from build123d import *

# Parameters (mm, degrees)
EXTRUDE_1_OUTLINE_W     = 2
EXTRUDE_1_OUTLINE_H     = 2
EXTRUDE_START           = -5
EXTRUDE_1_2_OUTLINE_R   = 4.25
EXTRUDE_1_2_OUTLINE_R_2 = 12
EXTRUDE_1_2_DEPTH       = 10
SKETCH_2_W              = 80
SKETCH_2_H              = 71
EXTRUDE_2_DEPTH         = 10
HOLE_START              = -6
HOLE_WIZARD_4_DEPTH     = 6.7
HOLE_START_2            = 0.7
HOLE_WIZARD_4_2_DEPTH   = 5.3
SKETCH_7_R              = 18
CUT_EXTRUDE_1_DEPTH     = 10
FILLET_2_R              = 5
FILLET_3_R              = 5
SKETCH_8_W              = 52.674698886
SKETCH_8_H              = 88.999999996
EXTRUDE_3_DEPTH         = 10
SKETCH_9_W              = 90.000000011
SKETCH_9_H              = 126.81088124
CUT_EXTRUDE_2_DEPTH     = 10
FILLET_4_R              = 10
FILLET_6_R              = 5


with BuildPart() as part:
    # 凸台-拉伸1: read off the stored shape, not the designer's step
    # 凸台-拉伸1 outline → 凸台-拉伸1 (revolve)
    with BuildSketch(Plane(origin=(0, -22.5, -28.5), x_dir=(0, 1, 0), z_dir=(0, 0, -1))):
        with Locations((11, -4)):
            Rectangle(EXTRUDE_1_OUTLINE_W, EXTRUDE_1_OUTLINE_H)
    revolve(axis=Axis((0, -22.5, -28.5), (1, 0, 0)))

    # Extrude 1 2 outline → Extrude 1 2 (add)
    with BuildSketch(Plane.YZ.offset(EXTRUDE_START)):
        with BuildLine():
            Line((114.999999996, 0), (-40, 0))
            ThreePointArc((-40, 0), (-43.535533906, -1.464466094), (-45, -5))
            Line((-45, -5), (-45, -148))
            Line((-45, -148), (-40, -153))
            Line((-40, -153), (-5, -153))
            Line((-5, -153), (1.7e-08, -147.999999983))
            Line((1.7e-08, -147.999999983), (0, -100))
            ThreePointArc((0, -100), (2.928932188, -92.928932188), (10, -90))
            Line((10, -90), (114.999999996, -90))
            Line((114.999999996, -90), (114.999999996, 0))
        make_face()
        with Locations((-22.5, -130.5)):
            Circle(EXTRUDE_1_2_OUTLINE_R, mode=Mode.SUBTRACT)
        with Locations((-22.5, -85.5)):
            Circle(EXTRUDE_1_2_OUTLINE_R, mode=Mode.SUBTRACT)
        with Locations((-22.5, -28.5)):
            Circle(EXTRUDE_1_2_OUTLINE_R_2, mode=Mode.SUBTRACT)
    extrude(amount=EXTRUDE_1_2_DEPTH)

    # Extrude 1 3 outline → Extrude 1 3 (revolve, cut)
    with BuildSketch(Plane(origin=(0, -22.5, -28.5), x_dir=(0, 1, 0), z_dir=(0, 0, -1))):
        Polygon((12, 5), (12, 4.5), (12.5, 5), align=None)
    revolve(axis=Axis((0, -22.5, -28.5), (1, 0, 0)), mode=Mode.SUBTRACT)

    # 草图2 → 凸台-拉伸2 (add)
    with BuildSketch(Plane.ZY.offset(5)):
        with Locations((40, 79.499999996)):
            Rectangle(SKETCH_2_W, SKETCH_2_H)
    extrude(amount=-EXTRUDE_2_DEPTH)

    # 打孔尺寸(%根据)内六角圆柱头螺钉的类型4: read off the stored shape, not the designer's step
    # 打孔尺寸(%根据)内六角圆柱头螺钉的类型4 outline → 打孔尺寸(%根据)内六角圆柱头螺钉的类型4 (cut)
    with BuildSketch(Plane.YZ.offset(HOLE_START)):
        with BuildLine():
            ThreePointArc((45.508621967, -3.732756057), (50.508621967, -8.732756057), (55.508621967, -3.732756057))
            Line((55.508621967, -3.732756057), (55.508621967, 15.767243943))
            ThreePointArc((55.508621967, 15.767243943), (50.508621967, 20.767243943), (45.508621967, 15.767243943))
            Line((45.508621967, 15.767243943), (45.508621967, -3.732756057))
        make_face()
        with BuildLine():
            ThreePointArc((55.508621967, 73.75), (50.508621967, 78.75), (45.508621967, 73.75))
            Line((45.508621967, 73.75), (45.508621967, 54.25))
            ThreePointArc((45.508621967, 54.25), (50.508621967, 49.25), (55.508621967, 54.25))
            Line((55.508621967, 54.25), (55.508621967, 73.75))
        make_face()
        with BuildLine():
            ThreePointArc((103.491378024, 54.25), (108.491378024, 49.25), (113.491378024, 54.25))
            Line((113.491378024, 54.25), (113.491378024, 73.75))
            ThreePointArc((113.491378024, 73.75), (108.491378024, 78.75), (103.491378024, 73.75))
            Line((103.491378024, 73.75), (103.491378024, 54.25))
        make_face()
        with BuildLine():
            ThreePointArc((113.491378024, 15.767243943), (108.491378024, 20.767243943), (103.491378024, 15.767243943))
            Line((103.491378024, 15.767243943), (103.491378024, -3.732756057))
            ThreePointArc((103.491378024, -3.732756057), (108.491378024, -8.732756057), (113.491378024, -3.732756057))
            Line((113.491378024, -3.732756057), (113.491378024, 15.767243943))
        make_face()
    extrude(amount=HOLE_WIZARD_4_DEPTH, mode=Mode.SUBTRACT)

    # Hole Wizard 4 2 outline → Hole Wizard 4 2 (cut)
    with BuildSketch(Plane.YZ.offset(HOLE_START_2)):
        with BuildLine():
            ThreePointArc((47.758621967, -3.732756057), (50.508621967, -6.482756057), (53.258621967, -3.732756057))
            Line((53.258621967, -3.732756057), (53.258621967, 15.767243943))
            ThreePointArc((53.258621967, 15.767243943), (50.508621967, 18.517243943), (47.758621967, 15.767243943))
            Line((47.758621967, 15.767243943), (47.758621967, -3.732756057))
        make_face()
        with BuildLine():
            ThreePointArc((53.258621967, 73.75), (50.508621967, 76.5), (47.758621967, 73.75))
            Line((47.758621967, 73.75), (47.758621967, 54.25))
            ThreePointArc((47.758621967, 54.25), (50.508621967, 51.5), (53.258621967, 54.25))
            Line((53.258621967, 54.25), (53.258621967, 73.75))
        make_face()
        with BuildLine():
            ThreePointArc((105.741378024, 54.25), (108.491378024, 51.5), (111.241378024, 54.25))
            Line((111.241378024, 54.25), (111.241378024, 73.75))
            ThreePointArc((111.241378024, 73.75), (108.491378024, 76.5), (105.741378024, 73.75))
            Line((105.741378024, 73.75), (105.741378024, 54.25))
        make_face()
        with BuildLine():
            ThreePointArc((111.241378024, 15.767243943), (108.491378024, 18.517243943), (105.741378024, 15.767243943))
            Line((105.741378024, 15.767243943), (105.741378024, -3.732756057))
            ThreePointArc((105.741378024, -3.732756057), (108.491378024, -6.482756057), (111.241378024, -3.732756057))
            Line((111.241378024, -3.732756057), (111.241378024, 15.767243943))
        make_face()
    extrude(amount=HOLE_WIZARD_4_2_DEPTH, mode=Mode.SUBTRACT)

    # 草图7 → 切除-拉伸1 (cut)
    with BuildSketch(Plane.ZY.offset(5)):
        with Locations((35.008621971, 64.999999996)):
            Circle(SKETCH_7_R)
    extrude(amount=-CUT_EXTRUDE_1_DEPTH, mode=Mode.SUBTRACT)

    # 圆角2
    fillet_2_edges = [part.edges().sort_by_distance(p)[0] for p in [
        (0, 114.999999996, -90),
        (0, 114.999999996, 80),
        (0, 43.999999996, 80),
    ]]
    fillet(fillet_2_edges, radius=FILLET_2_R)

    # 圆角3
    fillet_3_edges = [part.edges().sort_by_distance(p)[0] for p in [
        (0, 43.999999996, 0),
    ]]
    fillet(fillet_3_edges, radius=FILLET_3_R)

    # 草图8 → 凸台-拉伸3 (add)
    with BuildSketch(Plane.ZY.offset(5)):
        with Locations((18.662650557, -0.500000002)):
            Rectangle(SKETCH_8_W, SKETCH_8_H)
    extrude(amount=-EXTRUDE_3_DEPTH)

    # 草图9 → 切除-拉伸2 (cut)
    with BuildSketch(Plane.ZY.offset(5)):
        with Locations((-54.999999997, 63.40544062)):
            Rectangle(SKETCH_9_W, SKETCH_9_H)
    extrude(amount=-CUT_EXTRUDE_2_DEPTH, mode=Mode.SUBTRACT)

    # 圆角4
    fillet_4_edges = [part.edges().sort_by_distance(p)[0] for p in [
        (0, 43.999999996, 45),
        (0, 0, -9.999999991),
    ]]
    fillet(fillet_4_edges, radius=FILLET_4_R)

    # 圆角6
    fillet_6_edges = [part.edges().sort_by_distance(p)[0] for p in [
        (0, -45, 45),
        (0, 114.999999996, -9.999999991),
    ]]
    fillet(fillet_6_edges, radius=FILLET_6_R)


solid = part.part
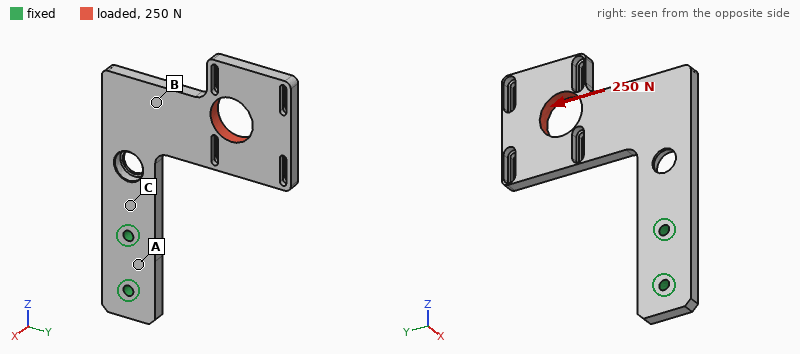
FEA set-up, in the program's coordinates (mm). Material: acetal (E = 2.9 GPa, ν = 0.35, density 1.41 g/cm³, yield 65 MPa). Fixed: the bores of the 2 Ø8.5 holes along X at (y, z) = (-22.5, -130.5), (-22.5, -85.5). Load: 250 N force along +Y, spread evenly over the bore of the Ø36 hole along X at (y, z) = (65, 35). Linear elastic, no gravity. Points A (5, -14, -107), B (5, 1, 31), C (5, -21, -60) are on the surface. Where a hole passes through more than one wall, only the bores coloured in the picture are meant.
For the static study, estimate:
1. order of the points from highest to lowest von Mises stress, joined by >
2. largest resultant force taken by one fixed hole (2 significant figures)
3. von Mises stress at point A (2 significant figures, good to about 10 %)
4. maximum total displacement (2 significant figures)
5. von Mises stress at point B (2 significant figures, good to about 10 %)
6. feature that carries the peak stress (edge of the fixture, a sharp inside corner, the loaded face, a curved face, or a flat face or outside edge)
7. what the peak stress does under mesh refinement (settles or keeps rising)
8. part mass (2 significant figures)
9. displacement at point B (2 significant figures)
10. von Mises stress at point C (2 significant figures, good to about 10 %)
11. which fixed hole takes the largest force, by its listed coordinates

A > C > B
740 N
2.7 MPa
2.4 mm
0.93 MPa
edge of the fixture
keeps rising
220 g
1.1 mm
1.9 MPa
(-22.5, -85.5)
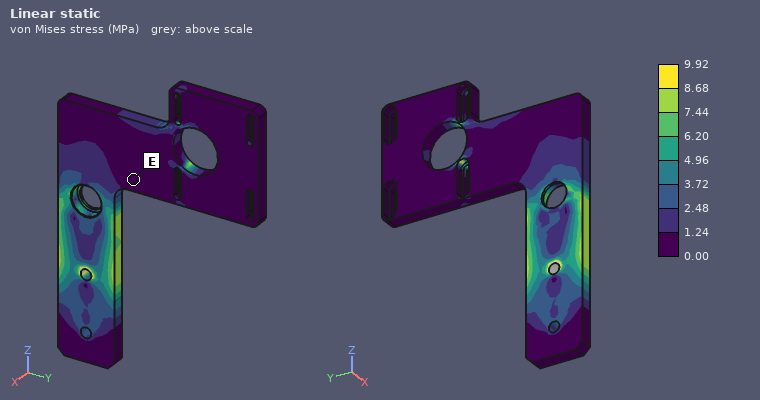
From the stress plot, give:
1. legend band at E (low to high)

0.00 to 1.24 MPa
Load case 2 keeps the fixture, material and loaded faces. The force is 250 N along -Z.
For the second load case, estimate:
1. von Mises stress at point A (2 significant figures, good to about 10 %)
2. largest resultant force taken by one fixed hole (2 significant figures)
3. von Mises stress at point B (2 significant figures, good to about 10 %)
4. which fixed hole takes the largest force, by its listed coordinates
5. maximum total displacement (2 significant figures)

2.2 MPa
420 N
1.5 MPa
(-22.5, -85.5)
2.5 mm
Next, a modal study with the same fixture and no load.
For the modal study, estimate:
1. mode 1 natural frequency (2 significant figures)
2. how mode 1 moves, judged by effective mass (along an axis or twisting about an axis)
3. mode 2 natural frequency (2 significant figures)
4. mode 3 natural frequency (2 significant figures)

42 Hz
along X
120 Hz
160 Hz
